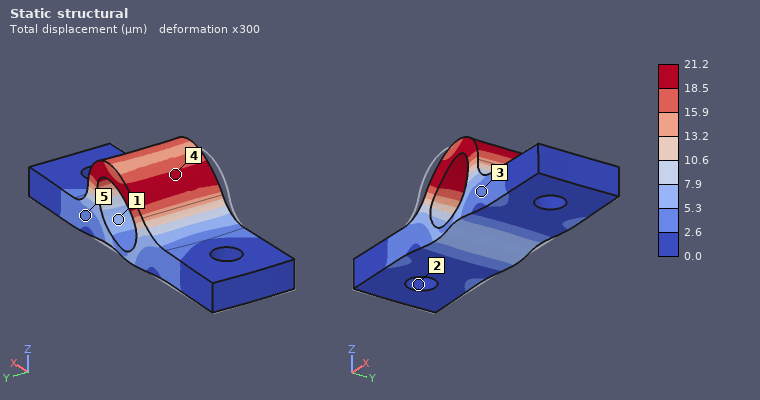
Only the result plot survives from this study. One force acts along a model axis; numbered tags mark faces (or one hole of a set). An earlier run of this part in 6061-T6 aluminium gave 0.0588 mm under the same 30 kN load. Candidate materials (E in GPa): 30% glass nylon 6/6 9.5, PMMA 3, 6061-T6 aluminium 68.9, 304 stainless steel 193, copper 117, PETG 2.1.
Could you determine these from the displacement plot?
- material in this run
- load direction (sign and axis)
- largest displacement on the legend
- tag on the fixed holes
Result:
304 stainless steel
+X
21.2 µm
2
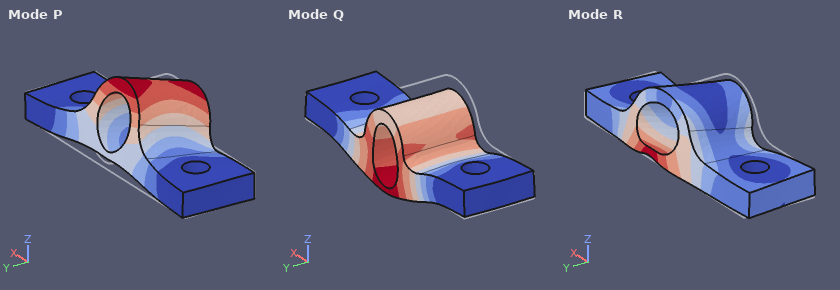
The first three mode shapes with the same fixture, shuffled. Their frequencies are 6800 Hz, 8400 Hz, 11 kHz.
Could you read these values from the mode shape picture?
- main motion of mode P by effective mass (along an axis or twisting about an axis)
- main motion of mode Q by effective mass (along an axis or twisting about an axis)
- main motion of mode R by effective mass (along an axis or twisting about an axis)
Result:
along Y
along Z
along Y
